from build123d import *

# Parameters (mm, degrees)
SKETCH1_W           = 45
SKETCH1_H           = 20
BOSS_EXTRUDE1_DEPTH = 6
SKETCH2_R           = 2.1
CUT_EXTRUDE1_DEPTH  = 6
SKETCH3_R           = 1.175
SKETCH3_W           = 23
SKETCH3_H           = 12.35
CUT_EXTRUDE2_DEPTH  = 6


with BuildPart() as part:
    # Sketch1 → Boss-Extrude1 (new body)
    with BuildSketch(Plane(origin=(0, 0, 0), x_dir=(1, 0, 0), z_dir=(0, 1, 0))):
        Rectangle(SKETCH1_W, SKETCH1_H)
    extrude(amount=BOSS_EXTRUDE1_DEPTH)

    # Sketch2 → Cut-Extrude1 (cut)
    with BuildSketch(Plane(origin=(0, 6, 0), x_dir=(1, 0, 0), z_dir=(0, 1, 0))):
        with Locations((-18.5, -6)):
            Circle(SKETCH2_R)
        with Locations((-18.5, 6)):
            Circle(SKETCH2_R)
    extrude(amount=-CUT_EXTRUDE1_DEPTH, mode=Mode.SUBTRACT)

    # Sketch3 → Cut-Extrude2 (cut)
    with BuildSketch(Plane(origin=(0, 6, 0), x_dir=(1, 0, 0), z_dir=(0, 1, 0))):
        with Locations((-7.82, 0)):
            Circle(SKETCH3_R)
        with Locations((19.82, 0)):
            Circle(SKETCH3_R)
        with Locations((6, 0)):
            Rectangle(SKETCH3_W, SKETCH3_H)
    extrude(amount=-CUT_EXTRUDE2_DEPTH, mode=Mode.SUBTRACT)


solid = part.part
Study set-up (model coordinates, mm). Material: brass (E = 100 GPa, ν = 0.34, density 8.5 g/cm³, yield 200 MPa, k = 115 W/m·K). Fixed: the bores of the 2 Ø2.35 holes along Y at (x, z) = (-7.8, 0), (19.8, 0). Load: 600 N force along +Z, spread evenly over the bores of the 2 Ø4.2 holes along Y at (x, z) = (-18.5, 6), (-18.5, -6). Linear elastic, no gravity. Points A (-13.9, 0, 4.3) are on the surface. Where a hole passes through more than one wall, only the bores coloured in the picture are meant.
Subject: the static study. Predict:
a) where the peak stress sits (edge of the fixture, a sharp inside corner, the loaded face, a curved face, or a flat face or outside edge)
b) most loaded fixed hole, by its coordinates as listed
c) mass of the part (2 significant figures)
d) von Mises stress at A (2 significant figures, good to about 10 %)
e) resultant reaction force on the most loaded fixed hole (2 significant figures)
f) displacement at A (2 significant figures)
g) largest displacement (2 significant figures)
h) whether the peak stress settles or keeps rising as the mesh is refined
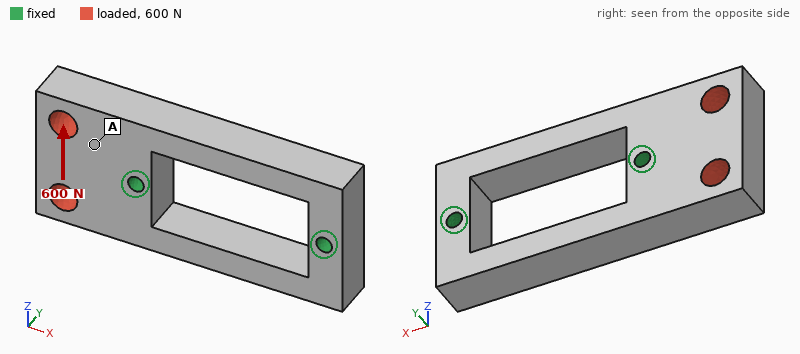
edge of the fixture
(-7.8, 0)
30 g
14 MPa
660 N
6.8 µm
17 µm
keeps rising
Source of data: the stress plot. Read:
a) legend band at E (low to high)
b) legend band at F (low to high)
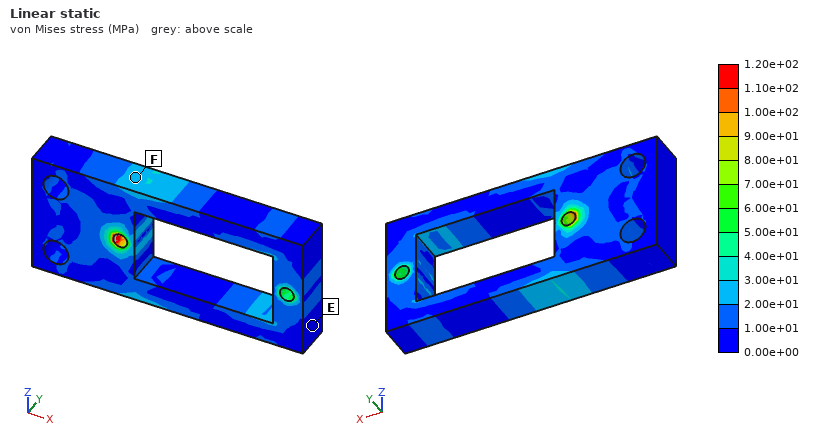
0.00e+00 to 1.00e+01 MPa
2.00e+01 to 3.00e+01 MPa
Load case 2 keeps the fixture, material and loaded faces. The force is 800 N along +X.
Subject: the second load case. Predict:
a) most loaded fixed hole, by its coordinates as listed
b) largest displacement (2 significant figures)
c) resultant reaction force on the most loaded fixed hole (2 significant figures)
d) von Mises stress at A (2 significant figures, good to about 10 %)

(-7.8, 0)
2.3 µm
730 N
7.6 MPa
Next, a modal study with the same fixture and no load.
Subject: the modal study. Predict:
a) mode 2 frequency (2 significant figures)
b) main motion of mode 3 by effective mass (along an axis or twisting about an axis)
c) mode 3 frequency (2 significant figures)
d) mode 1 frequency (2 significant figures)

11 kHz
twisting about X
13 kHz
9800 Hz
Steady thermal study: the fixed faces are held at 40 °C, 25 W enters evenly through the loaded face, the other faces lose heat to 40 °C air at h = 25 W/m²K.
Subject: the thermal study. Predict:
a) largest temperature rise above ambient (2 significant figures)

31 K
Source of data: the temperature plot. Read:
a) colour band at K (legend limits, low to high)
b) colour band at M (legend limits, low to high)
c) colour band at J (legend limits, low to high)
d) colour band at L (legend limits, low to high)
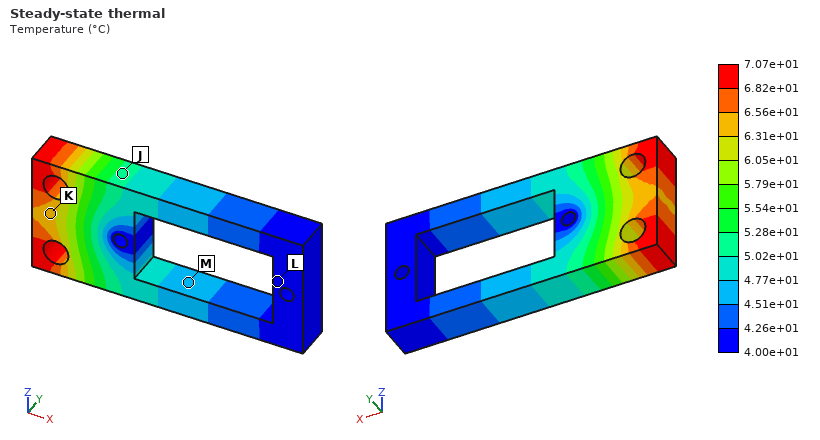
6.31e+01 to 6.56e+01 °C
4.51e+01 to 4.77e+01 °C
5.02e+01 to 5.28e+01 °C
4.00e+01 to 4.26e+01 °C
